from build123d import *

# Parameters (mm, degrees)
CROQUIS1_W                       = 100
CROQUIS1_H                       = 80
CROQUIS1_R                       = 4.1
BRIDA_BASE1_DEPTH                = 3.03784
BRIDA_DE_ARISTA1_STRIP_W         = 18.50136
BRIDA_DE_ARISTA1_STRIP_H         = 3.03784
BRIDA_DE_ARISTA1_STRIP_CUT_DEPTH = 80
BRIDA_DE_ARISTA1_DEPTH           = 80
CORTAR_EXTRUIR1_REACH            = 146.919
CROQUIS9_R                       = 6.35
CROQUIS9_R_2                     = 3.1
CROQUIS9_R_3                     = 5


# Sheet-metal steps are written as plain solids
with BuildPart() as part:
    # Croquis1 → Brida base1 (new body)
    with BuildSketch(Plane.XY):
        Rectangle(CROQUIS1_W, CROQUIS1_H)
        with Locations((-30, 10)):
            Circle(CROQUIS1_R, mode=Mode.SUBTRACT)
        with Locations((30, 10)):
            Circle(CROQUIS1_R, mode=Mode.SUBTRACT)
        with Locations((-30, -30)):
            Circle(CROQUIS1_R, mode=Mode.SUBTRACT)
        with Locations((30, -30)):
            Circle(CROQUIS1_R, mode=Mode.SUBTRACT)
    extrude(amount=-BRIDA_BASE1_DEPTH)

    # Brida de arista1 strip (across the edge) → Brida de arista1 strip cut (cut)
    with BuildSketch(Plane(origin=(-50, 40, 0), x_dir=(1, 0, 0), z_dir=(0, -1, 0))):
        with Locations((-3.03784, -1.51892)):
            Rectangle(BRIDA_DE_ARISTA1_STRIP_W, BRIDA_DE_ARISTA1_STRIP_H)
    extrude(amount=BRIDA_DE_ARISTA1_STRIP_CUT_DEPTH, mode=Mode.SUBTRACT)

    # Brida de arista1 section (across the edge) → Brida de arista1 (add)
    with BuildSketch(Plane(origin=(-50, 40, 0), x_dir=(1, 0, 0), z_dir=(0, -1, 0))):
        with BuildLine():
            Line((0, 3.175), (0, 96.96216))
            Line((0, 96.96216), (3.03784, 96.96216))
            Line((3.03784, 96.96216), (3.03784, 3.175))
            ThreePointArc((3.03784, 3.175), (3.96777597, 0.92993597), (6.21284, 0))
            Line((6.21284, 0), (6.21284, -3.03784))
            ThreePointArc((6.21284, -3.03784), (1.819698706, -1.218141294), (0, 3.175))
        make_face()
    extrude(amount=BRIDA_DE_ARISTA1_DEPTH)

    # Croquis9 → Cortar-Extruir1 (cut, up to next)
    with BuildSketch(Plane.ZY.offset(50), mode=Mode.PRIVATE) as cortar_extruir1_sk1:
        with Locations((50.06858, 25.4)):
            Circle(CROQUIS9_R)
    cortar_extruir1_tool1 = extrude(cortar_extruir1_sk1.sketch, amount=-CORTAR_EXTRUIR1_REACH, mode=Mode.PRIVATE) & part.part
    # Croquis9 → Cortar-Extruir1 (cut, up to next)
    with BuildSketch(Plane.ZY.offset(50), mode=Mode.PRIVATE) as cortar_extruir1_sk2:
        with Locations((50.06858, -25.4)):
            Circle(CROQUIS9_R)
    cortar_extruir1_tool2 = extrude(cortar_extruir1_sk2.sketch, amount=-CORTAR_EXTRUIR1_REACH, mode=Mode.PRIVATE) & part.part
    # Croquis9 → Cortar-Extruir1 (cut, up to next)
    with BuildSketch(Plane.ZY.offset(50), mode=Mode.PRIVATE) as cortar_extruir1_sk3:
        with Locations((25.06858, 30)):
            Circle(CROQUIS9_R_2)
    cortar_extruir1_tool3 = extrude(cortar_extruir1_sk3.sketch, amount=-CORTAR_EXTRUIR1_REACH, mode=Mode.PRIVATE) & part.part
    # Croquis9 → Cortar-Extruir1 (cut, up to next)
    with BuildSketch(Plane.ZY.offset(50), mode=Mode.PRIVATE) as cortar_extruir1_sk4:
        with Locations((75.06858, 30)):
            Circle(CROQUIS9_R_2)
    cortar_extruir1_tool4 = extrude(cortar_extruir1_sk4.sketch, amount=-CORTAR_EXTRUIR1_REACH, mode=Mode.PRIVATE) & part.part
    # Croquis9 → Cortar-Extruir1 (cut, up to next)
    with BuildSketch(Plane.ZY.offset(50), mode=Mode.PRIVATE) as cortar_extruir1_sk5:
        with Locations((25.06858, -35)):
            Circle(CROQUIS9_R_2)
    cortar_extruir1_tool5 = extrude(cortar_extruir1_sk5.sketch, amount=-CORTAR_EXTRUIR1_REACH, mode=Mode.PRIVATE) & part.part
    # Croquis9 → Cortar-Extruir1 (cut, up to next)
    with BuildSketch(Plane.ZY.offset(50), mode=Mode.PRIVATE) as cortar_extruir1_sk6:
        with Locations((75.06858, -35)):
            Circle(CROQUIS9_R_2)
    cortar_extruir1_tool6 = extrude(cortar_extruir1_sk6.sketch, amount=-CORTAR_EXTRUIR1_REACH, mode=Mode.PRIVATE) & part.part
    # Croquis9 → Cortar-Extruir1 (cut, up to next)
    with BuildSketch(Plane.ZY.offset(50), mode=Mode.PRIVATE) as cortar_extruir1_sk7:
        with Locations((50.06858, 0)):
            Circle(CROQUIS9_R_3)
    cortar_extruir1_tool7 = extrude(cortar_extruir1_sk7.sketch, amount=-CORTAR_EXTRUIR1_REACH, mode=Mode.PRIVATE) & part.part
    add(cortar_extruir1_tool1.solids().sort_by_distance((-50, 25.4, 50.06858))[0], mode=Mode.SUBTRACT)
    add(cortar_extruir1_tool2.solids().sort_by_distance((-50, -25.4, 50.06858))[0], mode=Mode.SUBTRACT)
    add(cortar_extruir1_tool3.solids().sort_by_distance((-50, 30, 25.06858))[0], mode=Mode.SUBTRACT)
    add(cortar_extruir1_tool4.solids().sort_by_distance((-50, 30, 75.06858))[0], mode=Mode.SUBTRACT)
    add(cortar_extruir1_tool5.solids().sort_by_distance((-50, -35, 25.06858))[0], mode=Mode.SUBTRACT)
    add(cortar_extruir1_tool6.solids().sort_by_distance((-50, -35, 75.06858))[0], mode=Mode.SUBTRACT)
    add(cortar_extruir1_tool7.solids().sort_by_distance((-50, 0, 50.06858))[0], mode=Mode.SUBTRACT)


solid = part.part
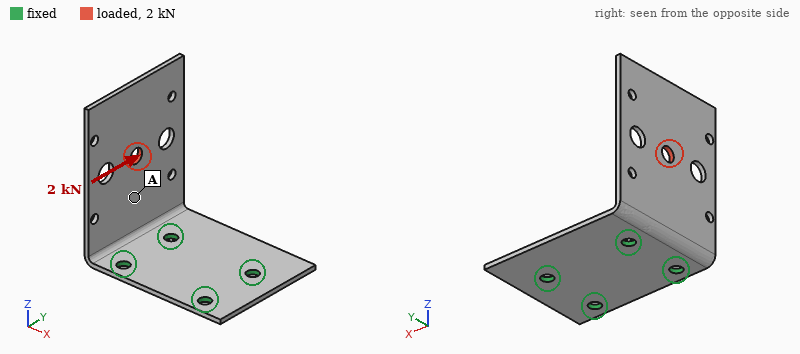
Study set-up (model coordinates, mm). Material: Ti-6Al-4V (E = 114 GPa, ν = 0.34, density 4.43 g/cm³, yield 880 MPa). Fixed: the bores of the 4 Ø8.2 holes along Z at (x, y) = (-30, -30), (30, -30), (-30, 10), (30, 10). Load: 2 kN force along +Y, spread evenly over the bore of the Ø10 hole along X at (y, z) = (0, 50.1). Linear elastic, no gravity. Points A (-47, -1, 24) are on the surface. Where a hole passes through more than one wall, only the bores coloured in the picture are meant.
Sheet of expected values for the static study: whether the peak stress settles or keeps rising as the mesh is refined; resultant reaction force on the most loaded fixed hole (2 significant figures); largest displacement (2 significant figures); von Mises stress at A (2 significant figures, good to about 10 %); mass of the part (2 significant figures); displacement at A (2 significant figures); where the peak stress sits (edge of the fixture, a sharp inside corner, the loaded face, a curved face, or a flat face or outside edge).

keeps rising
2.6 kN
1.5 mm
60 MPa
200 g
0.32 mm
edge of the fixture
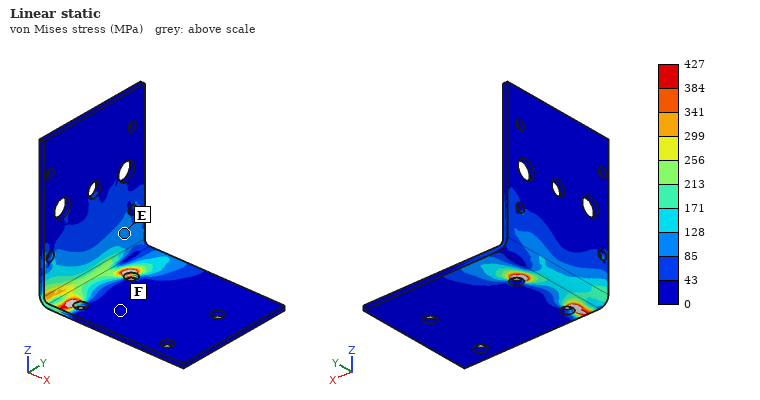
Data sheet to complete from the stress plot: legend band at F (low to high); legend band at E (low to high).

0 to 43 MPa
85 to 128 MPa
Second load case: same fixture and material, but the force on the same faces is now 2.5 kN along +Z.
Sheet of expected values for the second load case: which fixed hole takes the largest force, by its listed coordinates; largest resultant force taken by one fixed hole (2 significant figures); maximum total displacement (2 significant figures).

(-30, 10)
1.8 kN
1.8 mm
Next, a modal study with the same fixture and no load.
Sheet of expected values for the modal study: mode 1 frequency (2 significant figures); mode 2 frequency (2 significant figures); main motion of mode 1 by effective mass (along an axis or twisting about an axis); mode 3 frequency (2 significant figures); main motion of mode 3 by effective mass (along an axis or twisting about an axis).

210 Hz
630 Hz
along X
880 Hz
along Y
